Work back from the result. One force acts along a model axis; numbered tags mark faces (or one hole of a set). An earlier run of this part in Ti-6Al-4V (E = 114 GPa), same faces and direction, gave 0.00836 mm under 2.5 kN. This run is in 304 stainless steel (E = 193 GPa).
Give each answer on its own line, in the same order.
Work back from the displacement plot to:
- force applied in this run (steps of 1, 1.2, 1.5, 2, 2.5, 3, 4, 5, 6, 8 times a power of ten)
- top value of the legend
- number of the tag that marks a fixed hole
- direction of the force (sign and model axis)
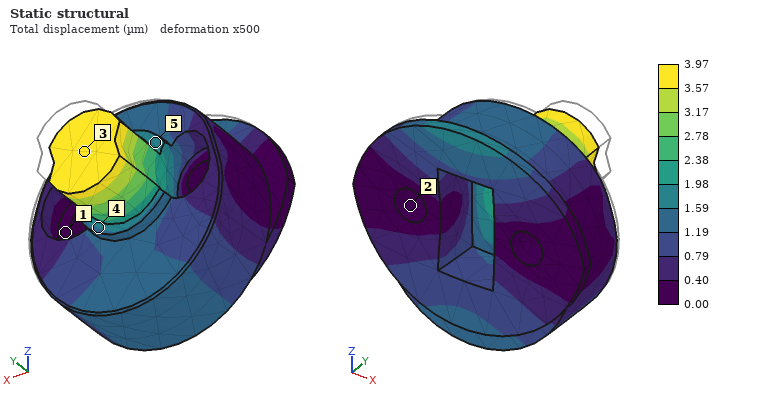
2 kN
3.97 µm
2
-Y
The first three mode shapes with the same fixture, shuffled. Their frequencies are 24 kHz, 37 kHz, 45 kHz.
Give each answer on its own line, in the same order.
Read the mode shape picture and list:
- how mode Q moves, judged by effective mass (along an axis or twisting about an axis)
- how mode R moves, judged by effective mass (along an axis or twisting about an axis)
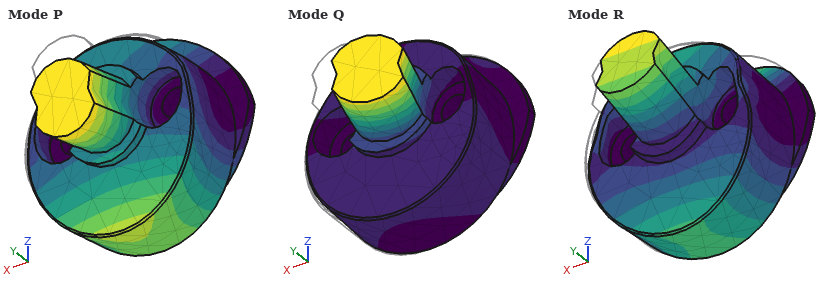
along X
along Y
